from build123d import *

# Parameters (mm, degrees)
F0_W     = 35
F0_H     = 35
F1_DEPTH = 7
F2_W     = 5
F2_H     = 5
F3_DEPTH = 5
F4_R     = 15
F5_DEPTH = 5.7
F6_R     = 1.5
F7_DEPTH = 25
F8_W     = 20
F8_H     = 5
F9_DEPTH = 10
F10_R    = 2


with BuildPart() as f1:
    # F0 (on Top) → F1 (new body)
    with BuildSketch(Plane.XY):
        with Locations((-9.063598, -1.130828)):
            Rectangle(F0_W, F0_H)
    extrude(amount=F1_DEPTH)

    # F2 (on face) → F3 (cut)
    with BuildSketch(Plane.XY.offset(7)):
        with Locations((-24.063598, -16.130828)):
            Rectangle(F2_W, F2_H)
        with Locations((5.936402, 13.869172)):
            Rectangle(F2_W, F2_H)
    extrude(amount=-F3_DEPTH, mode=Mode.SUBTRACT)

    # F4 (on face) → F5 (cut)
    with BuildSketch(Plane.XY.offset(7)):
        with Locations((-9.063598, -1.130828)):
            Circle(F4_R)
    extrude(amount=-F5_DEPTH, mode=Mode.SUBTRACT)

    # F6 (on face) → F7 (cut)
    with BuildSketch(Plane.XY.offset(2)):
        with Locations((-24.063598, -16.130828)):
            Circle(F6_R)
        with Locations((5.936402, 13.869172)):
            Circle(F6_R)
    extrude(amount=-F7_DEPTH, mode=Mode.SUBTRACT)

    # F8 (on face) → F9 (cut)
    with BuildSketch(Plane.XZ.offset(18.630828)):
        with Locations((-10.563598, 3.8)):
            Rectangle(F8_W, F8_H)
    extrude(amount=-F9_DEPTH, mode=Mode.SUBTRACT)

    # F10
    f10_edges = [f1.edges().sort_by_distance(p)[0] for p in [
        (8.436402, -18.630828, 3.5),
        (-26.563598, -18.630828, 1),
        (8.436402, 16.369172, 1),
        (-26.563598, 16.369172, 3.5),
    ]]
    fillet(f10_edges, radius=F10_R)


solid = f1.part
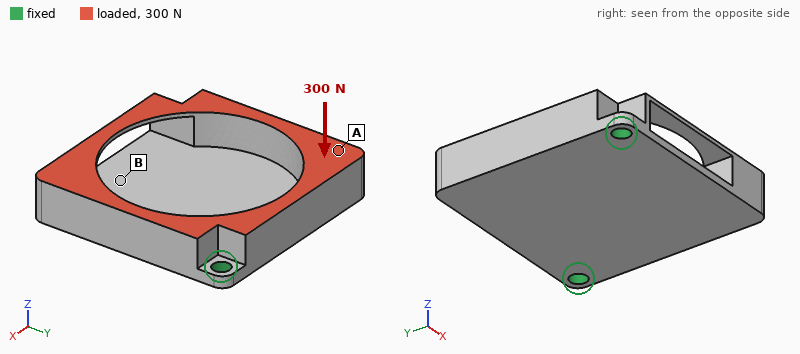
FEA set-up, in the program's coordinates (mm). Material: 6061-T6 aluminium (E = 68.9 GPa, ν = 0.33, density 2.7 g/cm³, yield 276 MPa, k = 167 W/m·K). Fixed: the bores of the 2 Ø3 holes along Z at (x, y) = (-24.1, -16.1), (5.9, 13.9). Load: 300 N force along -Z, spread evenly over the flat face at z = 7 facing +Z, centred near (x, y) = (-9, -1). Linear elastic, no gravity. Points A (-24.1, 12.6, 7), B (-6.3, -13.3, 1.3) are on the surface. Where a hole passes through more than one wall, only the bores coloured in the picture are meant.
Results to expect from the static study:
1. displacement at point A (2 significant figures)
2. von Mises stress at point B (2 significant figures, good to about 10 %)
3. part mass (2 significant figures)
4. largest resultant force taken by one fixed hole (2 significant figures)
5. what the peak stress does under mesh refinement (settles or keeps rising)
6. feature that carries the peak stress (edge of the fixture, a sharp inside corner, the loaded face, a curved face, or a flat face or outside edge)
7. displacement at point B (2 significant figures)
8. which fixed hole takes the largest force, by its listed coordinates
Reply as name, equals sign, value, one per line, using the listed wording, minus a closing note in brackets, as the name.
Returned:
displacement at point A = 0.052 mm
von Mises stress at point B = 33 MPa
part mass = 10 g
largest resultant force taken by one fixed hole = 180 N
what the peak stress does under mesh refinement = keeps rising
feature that carries the peak stress = edge of the fixture
displacement at point B = 0.099 mm
which fixed hole takes the largest force, by its listed coordinates = (5.9, 13.9)
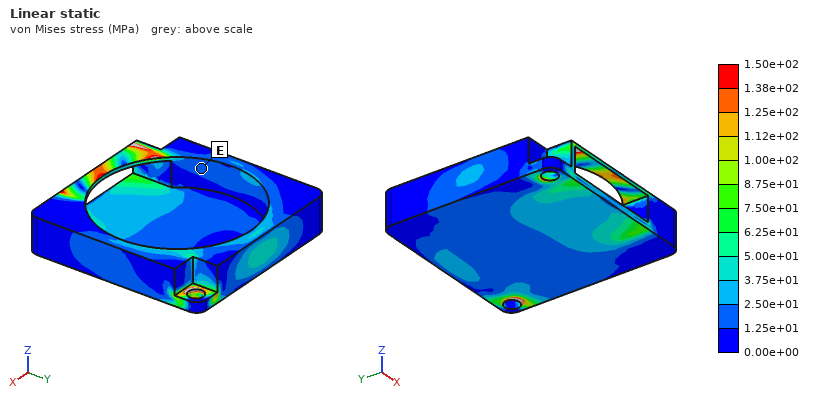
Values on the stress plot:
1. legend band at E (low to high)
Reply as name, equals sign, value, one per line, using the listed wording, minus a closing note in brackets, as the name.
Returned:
legend band at E = 1.25e+01 to 2.50e+01 MPa
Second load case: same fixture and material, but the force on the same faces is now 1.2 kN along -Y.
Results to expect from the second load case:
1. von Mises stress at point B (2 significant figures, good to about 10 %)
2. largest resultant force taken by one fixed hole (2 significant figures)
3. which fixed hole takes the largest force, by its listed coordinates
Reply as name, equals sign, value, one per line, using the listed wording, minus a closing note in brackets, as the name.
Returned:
von Mises stress at point B = 48 MPa
largest resultant force taken by one fixed hole = 650 N
which fixed hole takes the largest force, by its listed coordinates = (5.9, 13.9)
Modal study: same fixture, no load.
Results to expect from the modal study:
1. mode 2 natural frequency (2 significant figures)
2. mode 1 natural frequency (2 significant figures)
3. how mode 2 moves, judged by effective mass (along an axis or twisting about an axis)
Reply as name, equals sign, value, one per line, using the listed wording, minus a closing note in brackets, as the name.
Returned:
mode 2 natural frequency = 3600 Hz
mode 1 natural frequency = 2500 Hz
how mode 2 moves, judged by effective mass = along Z
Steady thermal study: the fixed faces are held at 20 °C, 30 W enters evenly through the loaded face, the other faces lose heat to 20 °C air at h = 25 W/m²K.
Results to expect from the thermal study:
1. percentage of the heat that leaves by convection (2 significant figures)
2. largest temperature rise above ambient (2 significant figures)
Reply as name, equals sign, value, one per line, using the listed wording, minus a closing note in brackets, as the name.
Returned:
percentage of the heat that leaves by convection = 6.8 %
largest temperature rise above ambient = 52 K
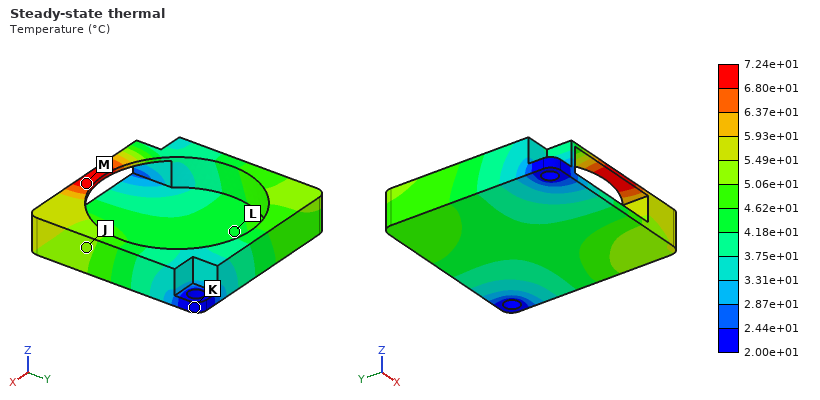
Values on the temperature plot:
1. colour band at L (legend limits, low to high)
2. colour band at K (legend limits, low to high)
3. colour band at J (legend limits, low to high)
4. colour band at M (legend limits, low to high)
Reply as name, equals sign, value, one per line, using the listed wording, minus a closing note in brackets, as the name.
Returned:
colour band at L = 4.18e+01 to 4.62e+01 °C
colour band at K = 2.00e+01 to 2.44e+01 °C
colour band at J = 5.06e+01 to 5.49e+01 °C
colour band at M = 6.80e+01 to 7.24e+01 °C
